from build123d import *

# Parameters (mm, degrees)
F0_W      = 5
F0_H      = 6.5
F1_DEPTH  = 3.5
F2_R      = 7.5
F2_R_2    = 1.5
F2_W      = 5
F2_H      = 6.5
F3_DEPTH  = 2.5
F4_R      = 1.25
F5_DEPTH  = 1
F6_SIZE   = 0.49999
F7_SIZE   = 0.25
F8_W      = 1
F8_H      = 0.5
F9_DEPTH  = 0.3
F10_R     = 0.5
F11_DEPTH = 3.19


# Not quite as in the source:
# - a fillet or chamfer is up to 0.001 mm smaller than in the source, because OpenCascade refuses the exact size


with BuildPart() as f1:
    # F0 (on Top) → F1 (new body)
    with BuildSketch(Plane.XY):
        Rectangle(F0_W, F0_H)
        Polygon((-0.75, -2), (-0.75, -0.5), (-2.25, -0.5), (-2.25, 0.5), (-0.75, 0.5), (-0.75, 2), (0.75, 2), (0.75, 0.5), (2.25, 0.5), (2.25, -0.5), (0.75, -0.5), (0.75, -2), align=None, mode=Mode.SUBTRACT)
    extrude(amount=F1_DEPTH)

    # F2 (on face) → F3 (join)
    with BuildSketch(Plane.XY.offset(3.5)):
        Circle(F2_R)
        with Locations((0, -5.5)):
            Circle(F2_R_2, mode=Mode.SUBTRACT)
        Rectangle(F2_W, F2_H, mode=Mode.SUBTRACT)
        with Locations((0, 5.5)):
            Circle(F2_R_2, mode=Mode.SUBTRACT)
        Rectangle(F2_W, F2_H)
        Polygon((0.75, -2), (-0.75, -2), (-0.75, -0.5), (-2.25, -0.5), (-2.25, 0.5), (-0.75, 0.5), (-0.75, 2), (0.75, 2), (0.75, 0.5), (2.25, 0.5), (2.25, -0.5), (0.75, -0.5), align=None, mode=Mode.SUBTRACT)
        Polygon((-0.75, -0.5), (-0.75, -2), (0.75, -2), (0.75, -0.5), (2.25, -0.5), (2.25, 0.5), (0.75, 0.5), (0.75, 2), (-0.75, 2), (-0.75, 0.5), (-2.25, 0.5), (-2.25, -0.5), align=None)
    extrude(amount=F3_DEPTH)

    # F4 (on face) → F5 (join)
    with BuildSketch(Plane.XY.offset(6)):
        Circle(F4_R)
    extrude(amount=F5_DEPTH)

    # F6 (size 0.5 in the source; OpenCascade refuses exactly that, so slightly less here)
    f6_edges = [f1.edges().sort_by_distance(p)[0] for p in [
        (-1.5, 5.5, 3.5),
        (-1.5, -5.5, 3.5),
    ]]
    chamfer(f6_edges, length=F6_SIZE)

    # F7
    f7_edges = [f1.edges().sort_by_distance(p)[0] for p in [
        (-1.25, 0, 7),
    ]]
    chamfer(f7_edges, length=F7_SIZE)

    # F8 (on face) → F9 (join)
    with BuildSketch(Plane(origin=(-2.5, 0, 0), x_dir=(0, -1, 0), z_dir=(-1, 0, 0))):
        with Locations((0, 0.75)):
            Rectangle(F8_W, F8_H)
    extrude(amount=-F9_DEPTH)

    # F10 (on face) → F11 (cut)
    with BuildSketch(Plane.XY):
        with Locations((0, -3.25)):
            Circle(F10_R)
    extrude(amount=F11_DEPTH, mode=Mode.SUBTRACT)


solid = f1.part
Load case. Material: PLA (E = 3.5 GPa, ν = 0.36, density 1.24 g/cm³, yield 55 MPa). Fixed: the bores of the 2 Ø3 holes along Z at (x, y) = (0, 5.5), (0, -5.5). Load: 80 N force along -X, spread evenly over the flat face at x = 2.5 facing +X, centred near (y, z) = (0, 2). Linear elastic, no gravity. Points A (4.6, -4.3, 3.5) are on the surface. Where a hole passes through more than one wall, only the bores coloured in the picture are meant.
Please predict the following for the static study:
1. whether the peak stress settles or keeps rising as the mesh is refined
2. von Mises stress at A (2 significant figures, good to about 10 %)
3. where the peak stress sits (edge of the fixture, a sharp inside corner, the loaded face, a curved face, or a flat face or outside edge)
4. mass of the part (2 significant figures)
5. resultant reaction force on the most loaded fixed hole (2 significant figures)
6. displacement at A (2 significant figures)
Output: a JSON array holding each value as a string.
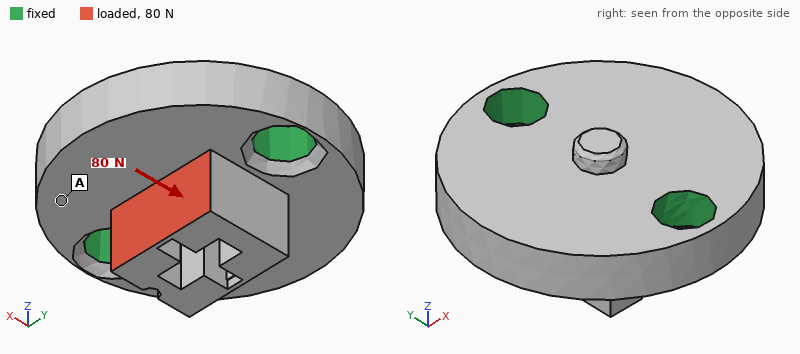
["keeps rising", "2.6 MPa", "edge of the fixture", "0.61 g", "40 N", "18 µm"]
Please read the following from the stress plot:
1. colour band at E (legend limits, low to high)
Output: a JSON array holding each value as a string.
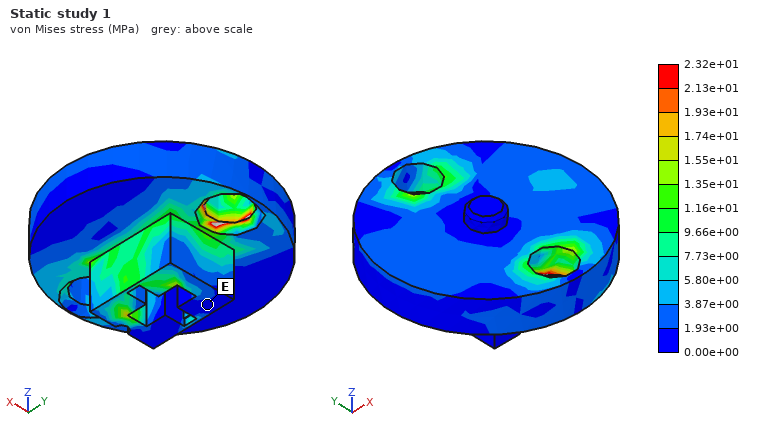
["0.00e+00 to 1.93e+00 MPa"]
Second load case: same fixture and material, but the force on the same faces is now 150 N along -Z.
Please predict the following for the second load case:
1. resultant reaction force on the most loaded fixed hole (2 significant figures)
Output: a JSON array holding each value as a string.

["79 N"]
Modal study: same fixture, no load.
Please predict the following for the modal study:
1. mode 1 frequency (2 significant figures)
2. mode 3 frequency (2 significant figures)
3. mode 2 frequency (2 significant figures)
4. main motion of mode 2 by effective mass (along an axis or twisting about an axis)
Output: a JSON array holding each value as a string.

["13 kHz", "31 kHz", "17 kHz", "along Z"]
